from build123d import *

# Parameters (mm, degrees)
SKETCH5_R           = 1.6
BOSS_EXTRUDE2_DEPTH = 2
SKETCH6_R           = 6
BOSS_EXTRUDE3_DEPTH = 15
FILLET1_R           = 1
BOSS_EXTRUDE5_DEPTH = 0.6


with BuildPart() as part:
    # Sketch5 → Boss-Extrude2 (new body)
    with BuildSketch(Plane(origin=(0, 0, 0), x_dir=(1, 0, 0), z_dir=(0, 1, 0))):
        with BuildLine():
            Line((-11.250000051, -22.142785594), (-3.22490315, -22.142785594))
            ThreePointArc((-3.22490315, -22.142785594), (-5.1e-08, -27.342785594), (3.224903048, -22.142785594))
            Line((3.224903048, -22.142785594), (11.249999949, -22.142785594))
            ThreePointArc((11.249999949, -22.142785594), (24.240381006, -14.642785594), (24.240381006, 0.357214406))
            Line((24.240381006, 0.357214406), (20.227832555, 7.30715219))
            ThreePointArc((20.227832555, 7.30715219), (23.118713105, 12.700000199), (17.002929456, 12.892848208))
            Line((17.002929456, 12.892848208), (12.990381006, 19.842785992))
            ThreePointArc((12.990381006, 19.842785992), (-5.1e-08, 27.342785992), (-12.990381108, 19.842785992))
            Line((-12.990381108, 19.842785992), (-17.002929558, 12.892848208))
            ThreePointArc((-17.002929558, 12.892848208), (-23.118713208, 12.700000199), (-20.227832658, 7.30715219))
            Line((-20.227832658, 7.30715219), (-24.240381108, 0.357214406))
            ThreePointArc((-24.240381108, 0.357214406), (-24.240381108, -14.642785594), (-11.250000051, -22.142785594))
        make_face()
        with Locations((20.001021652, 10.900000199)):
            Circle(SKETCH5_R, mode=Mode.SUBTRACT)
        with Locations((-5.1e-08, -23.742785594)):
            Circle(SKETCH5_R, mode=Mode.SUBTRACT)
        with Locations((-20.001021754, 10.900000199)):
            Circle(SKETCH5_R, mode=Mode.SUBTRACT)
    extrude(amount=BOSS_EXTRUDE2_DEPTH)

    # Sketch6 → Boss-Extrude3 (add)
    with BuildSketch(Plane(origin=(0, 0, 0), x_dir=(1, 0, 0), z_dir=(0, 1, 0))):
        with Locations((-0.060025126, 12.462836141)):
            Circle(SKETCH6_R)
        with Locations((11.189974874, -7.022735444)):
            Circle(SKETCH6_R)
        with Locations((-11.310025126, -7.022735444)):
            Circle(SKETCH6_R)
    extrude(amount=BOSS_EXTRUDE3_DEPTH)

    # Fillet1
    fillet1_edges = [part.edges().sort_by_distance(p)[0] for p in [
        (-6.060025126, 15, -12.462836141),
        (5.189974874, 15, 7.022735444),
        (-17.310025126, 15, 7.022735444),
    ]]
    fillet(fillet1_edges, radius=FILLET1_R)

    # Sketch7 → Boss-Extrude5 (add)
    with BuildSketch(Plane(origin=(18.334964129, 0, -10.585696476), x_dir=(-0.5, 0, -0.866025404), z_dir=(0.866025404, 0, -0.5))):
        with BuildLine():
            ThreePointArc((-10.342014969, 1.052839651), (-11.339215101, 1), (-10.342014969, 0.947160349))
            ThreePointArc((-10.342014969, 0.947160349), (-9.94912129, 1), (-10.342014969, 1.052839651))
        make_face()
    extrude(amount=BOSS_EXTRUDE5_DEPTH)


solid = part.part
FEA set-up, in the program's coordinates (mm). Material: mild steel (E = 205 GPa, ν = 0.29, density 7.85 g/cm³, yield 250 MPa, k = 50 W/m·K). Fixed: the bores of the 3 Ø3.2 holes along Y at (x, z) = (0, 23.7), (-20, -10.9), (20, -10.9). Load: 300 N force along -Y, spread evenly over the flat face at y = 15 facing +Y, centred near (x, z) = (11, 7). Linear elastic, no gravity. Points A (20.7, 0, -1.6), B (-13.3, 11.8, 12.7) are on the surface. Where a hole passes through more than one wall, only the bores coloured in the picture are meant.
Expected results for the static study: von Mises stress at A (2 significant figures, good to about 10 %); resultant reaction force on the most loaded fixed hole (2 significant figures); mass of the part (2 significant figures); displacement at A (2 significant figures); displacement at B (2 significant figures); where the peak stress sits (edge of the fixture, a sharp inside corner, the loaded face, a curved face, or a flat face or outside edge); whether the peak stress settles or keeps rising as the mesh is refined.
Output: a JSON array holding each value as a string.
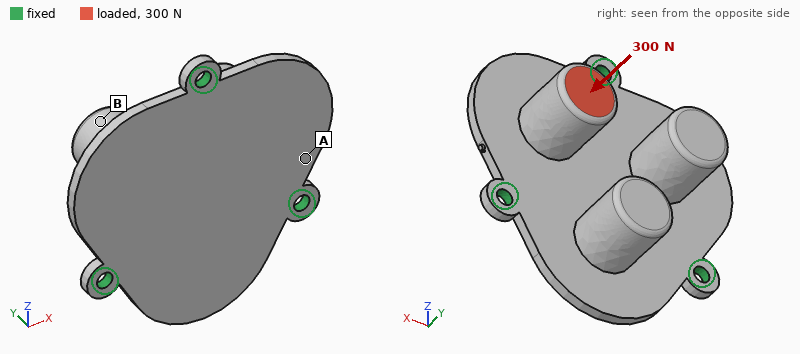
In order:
["33 MPa", "160 N", "66 g", "18 µm", "8.0 µm", "edge of the fixture", "keeps rising"]
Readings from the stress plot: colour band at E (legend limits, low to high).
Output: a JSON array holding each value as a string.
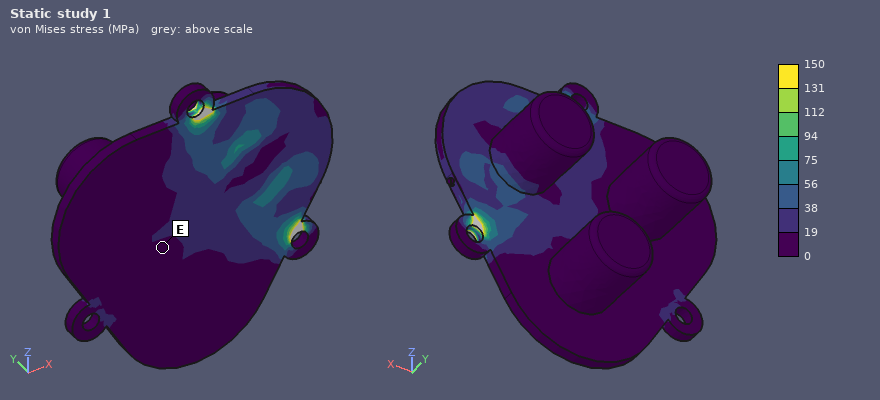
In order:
["0 to 19 MPa"]
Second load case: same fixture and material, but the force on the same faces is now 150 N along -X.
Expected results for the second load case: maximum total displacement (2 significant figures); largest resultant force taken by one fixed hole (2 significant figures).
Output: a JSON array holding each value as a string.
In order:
["39 µm", "77 N"]
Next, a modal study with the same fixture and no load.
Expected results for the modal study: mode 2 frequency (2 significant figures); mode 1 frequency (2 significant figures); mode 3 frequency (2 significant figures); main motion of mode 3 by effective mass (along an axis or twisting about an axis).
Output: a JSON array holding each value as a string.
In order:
["3100 Hz", "3100 Hz", "3600 Hz", "along Y"]
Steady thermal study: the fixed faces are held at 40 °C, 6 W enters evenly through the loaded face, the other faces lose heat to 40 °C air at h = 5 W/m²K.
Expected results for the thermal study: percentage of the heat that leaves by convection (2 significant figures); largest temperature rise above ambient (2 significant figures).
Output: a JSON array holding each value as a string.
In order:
["7.0 %", "43 K"]
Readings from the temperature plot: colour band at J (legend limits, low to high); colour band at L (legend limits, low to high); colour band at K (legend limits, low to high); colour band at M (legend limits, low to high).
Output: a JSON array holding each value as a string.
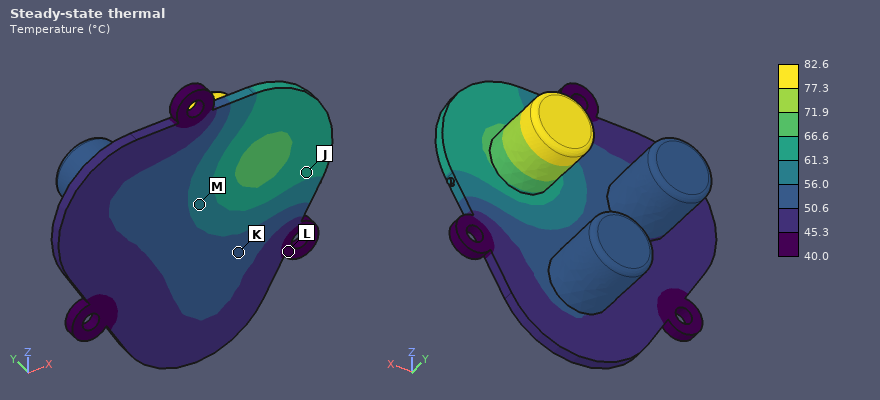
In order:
["61.3 to 66.6 °C", "40.0 to 45.3 °C", "50.6 to 56.0 °C", "56.0 to 61.3 °C"]
